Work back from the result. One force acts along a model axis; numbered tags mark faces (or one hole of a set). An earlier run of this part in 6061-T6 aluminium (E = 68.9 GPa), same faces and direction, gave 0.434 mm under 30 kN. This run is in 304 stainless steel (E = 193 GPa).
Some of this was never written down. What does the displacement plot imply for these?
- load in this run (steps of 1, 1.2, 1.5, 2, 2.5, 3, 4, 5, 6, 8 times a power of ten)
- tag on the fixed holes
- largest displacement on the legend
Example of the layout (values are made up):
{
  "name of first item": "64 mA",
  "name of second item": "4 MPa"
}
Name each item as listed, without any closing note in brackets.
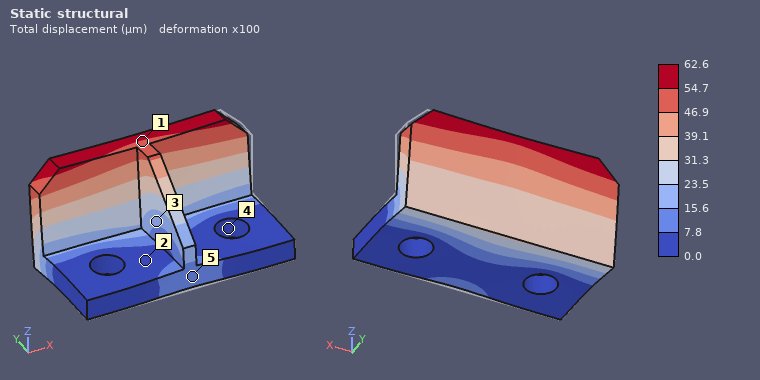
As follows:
{
  "load in this run": "12 kN",
  "tag on the fixed holes": "4",
  "largest displacement on the legend": "62.6 µm"
}
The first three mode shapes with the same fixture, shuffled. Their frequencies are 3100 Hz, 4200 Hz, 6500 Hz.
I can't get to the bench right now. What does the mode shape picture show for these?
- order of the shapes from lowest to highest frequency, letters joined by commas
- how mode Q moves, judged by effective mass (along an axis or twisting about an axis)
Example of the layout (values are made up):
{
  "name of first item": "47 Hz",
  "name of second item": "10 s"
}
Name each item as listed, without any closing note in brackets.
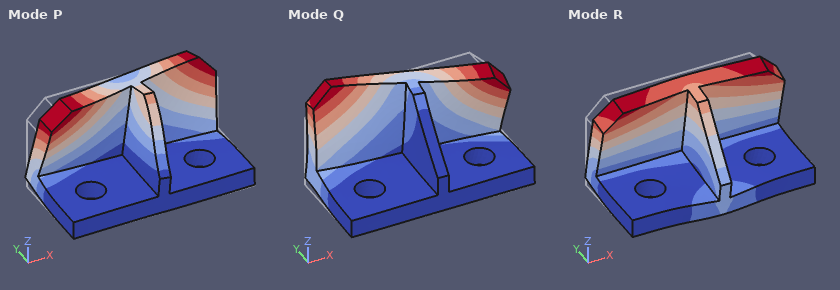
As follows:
{
  "order of the shapes from lowest to highest frequency, letters joined by commas": "R, P, Q",
  "how mode Q moves, judged by effective mass": "along X"
}
